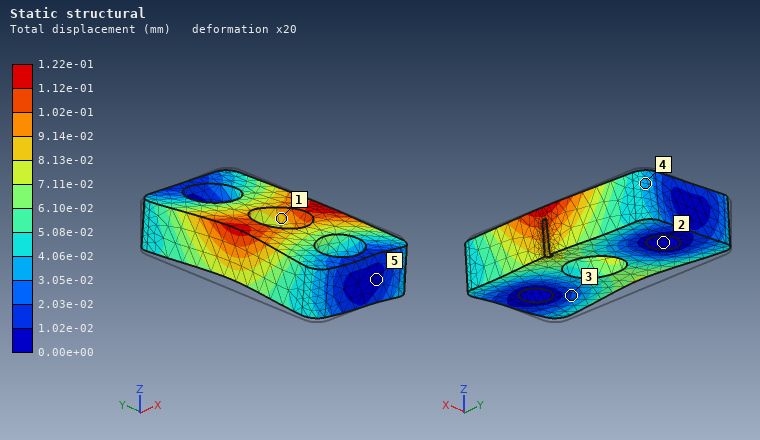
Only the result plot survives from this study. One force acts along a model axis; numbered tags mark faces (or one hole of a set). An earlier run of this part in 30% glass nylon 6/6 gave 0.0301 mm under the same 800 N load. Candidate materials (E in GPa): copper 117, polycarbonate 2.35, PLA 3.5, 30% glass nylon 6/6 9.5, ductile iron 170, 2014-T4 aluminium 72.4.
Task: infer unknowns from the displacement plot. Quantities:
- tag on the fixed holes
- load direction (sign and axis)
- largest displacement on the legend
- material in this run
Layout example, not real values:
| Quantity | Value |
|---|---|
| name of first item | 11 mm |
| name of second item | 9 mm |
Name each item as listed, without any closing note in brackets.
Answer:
| Quantity | Value |
|---|---|
| tag on the fixed holes | 2 |
| load direction | +X |
| largest displacement on the legend | 1.22e-01 mm |
| material in this run | polycarbonate |
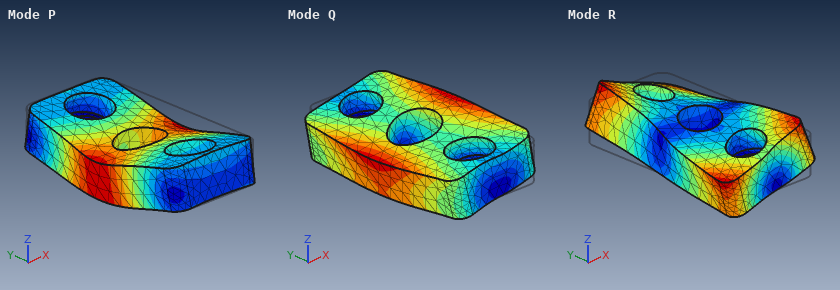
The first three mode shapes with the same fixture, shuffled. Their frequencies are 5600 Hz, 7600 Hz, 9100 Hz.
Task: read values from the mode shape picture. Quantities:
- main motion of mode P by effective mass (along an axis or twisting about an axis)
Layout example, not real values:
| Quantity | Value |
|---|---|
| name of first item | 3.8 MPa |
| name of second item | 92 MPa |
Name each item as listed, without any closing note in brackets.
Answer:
| Quantity | Value |
|---|---|
| main motion of mode P by effective mass | along Z |
